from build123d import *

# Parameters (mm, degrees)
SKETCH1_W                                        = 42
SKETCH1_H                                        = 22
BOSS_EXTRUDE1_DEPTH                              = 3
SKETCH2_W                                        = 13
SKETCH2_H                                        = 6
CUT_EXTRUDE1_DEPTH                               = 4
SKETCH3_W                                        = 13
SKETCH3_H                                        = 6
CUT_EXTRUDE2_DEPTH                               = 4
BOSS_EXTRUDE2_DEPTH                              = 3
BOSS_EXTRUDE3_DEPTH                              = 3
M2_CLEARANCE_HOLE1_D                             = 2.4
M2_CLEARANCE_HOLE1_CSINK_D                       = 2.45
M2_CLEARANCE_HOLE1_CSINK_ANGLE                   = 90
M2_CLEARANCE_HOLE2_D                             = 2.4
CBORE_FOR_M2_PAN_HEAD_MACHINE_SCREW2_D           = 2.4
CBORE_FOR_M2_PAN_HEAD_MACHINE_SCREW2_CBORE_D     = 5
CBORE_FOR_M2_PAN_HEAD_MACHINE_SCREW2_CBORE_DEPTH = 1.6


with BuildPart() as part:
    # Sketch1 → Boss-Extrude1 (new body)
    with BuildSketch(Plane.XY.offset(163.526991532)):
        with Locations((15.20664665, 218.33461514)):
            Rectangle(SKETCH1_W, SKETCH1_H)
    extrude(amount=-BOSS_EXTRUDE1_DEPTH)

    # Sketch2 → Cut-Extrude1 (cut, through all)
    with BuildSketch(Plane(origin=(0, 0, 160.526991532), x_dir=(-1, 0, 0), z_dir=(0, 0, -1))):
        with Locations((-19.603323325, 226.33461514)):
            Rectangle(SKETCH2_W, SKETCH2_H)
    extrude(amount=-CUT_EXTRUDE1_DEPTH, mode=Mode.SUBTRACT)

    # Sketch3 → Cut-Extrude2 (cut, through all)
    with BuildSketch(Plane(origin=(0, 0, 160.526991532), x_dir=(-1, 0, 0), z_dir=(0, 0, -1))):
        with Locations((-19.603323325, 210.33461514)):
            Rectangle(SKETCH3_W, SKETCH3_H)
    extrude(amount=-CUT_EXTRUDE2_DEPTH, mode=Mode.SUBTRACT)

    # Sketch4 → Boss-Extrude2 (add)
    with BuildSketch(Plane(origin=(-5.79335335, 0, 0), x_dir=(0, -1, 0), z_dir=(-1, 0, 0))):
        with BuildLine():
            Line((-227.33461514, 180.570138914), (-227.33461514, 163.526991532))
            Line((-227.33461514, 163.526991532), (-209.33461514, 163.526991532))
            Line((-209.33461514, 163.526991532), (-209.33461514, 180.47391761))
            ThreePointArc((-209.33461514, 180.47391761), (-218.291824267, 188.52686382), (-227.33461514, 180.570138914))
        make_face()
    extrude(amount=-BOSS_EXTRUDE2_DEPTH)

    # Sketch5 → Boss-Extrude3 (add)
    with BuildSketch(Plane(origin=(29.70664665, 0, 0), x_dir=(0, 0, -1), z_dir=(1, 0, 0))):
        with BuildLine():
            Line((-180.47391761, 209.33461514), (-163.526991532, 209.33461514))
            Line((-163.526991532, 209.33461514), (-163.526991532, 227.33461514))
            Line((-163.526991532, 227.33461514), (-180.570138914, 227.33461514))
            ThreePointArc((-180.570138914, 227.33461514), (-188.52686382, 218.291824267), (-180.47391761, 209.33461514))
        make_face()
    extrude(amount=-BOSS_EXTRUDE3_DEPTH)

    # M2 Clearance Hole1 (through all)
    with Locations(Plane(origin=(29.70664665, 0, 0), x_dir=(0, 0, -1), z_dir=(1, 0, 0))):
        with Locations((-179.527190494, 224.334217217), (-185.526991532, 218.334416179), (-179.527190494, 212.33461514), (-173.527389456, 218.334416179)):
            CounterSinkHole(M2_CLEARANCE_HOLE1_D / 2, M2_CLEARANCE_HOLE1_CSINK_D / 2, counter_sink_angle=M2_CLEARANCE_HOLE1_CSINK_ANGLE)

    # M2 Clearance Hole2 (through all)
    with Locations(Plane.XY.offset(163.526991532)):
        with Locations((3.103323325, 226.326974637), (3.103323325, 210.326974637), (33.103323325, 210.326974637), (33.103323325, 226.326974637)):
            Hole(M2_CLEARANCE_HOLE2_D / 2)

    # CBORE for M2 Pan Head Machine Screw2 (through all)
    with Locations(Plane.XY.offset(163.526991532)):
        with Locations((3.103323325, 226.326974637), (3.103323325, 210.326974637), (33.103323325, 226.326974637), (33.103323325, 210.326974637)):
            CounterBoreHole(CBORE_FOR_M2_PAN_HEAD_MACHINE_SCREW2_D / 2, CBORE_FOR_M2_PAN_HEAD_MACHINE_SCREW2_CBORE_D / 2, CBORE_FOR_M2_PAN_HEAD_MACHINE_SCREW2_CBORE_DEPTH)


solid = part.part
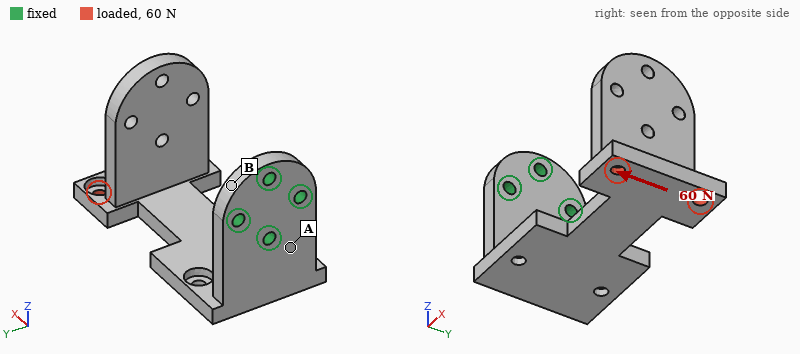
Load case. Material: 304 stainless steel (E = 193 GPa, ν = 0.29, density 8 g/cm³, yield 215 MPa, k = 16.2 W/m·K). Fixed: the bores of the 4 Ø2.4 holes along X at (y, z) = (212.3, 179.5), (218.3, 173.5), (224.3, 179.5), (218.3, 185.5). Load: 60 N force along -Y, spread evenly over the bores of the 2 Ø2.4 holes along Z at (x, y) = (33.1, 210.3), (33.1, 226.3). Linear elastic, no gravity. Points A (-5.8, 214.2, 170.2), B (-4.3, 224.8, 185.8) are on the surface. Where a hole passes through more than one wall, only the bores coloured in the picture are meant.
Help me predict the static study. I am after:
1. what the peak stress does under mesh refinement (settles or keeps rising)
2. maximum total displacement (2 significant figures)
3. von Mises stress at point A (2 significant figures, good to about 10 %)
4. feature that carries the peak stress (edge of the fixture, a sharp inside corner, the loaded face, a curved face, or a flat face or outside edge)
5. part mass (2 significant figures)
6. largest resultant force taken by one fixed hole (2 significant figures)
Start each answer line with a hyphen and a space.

- keeps rising
- 88 µm
- 50 MPa
- edge of the fixture
- 36 g
- 81 N
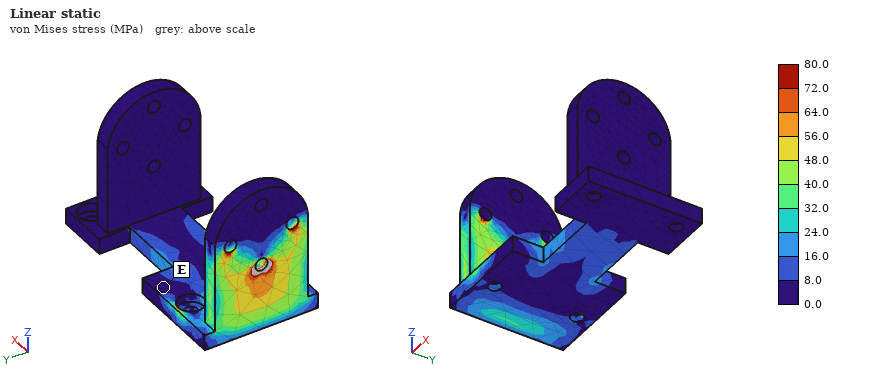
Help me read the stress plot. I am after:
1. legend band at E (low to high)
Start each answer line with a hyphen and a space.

- 0.0 to 8.0 MPa
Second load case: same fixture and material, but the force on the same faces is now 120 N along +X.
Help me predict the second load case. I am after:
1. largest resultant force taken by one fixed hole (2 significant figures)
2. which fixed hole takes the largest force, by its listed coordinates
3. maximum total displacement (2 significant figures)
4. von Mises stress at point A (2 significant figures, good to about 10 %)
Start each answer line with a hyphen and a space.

- 200 N
- (218.3, 173.5)
- 62 µm
- 35 MPa
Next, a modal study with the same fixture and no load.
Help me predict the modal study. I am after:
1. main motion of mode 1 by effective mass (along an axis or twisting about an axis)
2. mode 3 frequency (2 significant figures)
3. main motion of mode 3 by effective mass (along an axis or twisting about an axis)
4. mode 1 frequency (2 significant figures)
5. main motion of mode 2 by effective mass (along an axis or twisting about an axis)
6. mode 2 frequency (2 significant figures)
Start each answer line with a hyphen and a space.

- along Z
- 2000 Hz
- along X
- 640 Hz
- along Y
- 1000 Hz
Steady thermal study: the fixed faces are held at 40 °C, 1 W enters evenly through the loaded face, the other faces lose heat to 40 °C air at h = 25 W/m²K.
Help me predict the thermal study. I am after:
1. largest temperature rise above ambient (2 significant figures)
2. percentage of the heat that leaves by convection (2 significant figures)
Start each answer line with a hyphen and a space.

- 27 K
- 85 %
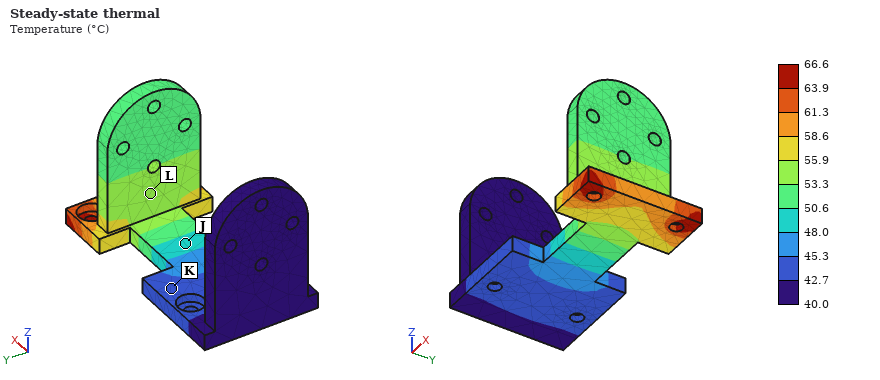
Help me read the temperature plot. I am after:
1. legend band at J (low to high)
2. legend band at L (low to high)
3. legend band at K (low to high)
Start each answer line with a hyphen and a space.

- 48.0 to 50.6 °C
- 53.3 to 55.9 °C
- 42.7 to 45.3 °C
